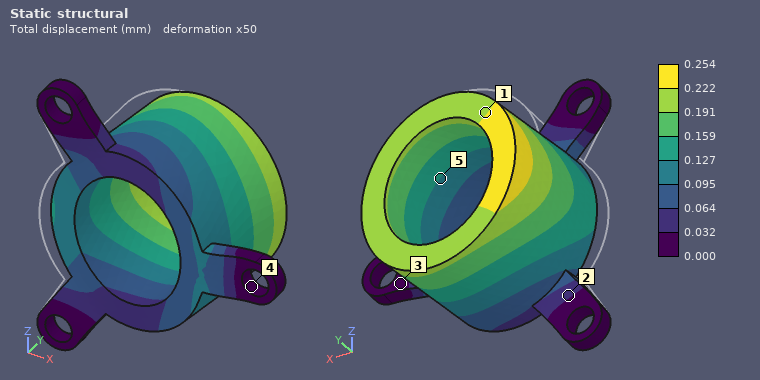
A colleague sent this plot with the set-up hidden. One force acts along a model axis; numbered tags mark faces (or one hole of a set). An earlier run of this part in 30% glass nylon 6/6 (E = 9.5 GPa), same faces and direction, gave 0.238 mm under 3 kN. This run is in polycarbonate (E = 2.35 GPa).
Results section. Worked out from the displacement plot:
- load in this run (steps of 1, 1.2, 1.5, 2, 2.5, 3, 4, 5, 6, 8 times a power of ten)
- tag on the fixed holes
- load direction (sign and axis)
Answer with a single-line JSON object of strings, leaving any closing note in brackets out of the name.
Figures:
{"load in this run": "800 N", "tag on the fixed holes": "4", "load direction": "+X"}
